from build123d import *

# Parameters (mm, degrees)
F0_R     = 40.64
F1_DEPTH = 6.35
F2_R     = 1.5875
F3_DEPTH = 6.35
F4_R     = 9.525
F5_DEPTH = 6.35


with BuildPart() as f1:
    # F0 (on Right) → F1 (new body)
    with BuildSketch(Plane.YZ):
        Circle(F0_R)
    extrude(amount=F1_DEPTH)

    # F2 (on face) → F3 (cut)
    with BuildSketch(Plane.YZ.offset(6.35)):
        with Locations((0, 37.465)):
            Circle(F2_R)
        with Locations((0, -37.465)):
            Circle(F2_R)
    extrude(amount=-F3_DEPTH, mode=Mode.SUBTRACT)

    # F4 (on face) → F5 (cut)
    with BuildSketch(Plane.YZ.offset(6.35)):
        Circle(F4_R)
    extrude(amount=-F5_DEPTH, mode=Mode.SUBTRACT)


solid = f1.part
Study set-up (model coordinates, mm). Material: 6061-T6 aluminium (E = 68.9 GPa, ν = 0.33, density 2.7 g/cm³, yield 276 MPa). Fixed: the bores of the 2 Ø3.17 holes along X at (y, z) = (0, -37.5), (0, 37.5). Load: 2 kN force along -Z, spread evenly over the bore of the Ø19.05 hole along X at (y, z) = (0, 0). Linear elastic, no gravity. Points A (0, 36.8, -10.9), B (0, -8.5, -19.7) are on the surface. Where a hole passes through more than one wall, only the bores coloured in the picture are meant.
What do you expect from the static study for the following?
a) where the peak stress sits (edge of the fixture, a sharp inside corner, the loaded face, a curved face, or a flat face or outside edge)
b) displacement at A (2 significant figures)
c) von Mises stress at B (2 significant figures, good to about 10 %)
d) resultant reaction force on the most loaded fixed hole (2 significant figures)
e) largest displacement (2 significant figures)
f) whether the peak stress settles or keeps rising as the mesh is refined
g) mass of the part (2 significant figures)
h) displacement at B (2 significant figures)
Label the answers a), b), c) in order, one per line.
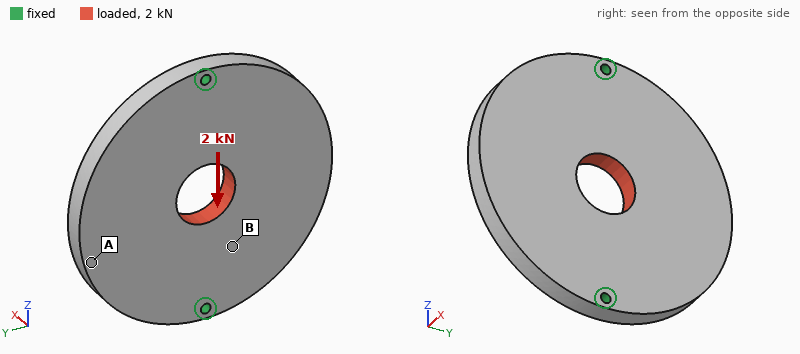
a) edge of the fixture
b) 2.7 µm
c) 5.3 MPa
d) 1.0 kN
e) 4.2 µm
f) keeps rising
g) 84 g
h) 2.9 µm
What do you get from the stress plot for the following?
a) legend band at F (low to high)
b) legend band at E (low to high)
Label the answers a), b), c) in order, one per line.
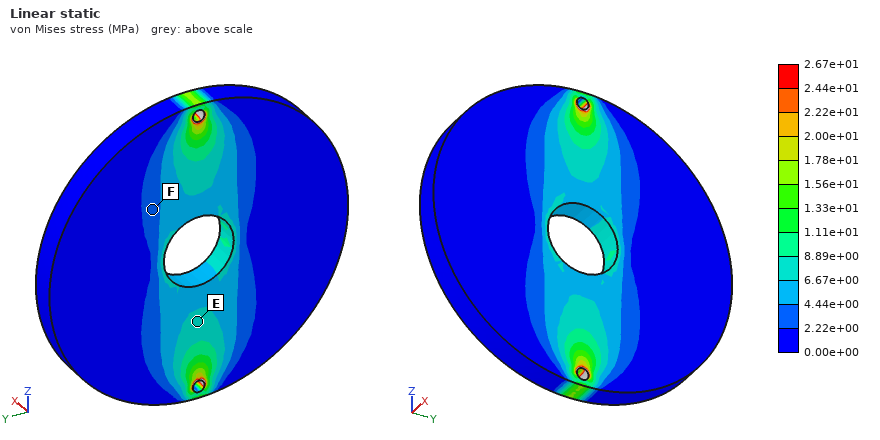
a) 2.22e+00 to 4.44e+00 MPa
b) 6.67e+00 to 8.89e+00 MPa
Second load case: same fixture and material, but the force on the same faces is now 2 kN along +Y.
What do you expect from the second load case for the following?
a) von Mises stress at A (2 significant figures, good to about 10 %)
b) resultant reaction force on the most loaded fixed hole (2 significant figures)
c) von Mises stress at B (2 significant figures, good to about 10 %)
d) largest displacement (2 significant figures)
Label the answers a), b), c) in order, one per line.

a) 3.8 MPa
b) 1.0 kN
c) 4.3 MPa
d) 5.9 µm
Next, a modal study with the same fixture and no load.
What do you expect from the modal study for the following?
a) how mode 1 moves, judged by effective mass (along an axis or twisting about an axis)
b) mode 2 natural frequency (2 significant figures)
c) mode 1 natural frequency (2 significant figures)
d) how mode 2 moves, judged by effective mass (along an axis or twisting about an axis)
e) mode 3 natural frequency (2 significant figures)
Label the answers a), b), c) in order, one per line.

a) twisting about Z
b) 2800 Hz
c) 2000 Hz
d) along X
e) 6500 Hz
